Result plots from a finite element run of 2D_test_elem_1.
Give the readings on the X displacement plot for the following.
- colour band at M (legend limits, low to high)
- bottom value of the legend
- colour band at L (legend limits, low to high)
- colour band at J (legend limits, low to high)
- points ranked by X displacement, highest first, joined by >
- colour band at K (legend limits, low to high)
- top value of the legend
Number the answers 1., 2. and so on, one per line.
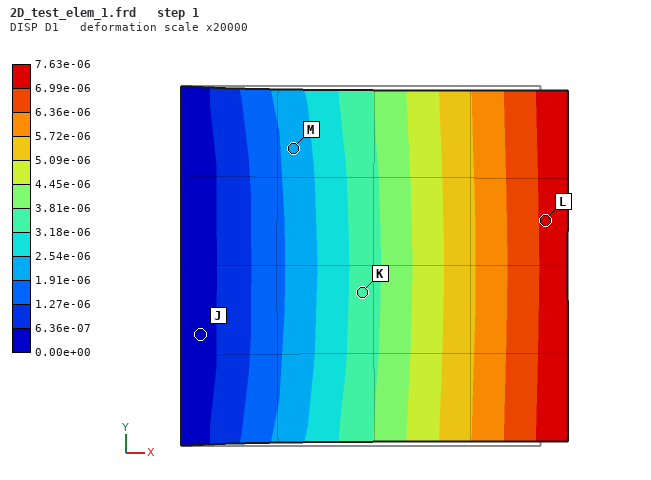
1. 1.91e-06 to 2.54e-06
2. 0.00e+00
3. 6.99e-06 to 7.63e-06
4. 0.00e+00 to 6.36e-07
5. L > K > M > J
6. 3.18e-06 to 3.81e-06
7. 7.63e-06
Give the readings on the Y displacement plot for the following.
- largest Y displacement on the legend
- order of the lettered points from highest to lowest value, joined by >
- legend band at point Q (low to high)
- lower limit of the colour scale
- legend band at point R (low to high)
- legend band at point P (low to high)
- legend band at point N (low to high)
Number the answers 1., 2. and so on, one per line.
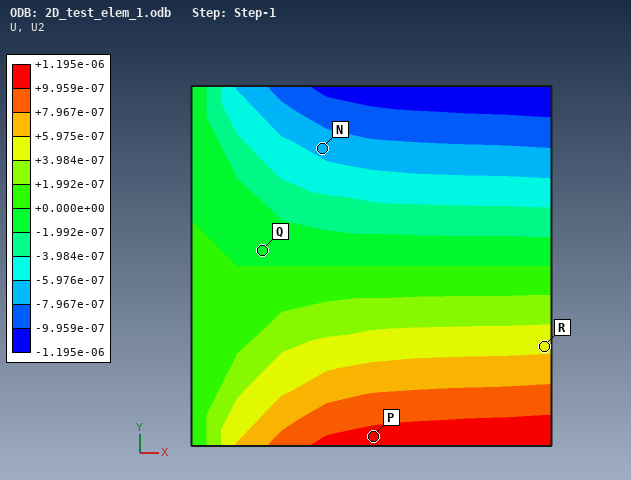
1. +1.195e-06
2. P > R > Q > N
3. -1.992e-07 to +0.000e+00
4. -1.195e-06
5. +3.984e-07 to +5.975e-07
6. +9.959e-07 to +1.195e-06
7. -7.967e-07 to -5.976e-07
